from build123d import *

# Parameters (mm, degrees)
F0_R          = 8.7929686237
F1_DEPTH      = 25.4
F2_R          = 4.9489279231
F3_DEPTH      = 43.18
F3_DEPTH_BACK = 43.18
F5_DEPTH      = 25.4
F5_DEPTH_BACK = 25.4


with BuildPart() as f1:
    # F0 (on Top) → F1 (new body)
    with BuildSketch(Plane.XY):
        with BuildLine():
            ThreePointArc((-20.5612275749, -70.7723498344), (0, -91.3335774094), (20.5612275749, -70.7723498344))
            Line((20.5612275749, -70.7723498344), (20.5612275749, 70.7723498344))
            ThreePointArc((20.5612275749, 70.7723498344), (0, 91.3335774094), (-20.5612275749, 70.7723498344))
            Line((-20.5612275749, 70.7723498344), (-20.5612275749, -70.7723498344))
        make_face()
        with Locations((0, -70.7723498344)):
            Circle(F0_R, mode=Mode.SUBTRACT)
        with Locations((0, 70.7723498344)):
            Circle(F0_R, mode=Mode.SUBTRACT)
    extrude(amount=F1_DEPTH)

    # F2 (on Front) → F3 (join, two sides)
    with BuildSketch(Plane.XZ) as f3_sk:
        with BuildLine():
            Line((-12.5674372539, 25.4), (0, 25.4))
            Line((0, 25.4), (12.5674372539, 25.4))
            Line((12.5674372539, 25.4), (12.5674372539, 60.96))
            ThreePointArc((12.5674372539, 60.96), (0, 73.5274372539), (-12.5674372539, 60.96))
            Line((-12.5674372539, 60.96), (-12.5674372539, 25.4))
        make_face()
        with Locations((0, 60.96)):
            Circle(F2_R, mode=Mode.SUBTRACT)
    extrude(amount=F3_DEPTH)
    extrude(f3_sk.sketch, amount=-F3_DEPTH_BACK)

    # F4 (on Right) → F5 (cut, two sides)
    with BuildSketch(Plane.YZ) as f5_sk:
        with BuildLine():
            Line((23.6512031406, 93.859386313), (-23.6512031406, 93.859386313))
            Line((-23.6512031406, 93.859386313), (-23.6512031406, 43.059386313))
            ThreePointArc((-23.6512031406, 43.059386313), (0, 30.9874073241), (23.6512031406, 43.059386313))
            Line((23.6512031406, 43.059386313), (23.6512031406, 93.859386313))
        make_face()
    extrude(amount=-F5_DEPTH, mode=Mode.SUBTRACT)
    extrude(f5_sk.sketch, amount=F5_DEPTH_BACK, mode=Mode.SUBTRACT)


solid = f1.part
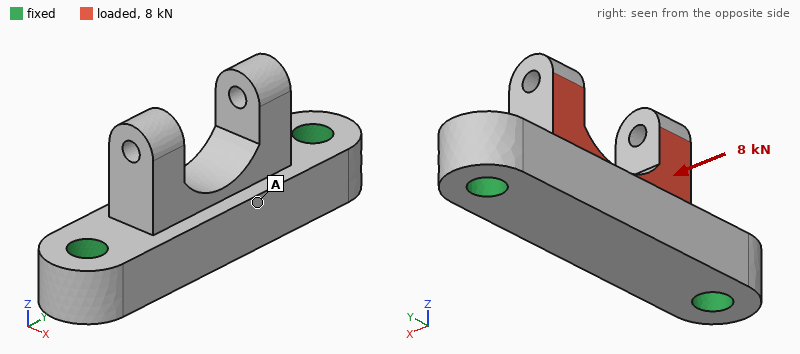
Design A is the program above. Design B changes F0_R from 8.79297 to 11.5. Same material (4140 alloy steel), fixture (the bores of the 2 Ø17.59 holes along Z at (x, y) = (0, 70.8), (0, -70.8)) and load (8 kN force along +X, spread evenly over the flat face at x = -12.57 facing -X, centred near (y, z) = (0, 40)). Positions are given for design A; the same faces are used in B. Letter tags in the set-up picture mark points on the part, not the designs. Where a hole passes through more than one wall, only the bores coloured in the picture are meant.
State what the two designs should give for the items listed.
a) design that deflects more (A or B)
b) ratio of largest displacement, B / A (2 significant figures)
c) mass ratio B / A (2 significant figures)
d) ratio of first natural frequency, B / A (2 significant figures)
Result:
A
0.89
0.96
1.1
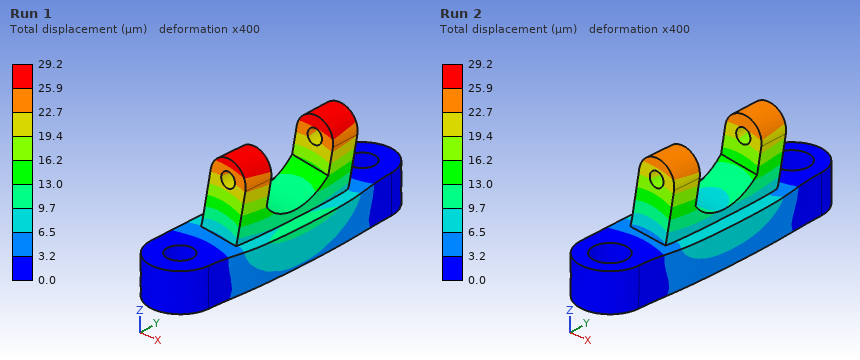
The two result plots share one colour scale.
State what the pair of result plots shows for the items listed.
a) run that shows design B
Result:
Run 2
